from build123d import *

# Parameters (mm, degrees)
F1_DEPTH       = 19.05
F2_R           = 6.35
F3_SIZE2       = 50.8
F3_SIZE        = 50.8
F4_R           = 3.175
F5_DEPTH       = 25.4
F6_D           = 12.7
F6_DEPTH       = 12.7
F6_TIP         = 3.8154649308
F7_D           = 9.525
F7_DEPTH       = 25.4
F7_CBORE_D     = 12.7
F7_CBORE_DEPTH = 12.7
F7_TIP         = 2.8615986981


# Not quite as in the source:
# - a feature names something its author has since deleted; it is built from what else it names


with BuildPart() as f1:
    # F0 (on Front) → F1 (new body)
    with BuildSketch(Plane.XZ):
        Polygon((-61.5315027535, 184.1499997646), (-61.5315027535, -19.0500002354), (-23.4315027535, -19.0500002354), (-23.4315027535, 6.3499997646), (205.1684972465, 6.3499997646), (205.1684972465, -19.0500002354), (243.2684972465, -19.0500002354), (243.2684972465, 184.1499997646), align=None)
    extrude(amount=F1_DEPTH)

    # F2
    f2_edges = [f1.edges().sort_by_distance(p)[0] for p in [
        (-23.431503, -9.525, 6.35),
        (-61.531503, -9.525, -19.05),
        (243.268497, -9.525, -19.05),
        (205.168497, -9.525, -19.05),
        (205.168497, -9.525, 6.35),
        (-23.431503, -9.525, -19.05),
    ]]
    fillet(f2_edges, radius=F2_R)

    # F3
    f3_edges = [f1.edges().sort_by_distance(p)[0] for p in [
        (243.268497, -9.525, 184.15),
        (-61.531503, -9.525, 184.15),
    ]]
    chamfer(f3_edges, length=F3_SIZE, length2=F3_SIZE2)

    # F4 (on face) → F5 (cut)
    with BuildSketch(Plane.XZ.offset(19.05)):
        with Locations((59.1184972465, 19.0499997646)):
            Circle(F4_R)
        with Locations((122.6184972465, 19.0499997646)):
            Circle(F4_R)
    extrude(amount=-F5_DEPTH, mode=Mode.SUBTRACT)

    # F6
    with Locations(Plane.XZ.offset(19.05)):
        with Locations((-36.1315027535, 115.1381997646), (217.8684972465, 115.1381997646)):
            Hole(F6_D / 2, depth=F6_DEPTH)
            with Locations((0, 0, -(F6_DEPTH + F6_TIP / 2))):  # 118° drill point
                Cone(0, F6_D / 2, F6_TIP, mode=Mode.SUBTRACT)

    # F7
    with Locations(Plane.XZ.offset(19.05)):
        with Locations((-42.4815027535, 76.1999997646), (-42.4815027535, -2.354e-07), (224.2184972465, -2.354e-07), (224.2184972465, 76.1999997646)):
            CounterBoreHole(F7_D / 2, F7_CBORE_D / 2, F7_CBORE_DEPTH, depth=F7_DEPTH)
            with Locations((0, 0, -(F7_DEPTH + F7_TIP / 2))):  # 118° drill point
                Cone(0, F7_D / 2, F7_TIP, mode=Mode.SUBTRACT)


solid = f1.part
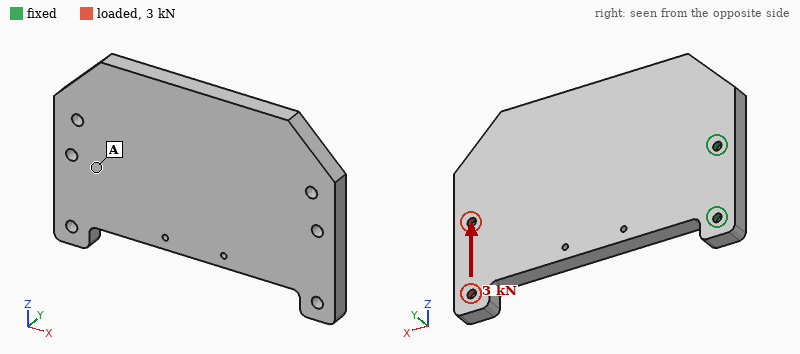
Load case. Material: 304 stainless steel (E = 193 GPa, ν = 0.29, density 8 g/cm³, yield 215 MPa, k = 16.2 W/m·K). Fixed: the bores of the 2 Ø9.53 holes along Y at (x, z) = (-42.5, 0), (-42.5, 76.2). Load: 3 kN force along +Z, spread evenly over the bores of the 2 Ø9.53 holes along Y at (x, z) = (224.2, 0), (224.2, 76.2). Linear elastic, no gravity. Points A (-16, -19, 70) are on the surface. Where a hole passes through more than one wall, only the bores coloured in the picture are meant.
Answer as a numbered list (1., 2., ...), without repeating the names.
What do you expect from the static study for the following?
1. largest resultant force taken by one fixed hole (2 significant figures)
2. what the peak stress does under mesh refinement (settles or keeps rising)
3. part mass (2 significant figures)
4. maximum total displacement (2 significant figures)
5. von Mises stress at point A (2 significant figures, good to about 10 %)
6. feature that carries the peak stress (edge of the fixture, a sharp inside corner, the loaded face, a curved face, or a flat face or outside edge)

1. 10 kN
2. keeps rising
3. 8.1 kg
4. 0.10 mm
5. 7.9 MPa
6. edge of the fixture
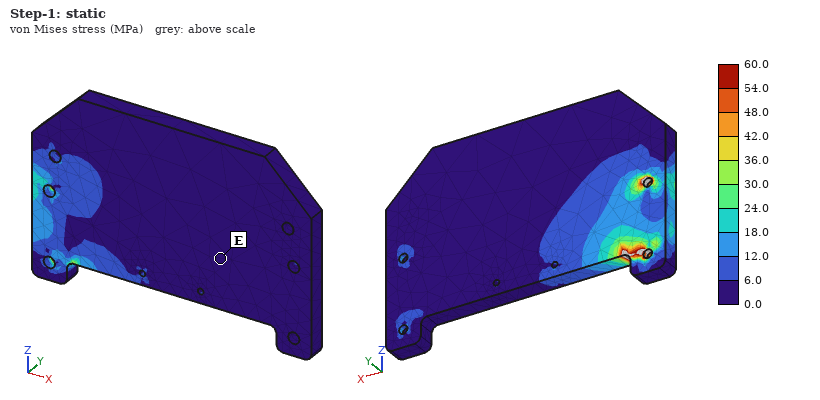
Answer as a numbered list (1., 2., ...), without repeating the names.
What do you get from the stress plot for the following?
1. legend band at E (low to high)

1. 0.0 to 6.0 MPa
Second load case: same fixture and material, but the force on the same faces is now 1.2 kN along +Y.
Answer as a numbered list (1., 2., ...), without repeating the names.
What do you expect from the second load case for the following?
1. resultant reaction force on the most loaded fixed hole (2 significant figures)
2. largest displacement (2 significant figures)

1. 1.6 kN
2. 1.1 mm
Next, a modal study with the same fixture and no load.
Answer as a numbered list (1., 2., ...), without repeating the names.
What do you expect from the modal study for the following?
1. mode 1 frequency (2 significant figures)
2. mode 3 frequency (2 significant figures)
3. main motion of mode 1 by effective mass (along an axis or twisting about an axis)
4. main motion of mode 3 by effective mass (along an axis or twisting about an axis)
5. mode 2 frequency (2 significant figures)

1. 110 Hz
2. 590 Hz
3. along Y
4. along Z
5. 450 Hz
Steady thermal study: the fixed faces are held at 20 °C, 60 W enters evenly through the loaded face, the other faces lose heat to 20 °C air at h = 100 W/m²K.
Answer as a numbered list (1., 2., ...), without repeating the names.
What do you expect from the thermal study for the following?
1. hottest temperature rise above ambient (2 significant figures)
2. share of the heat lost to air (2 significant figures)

1. 81 K
2. 100 %
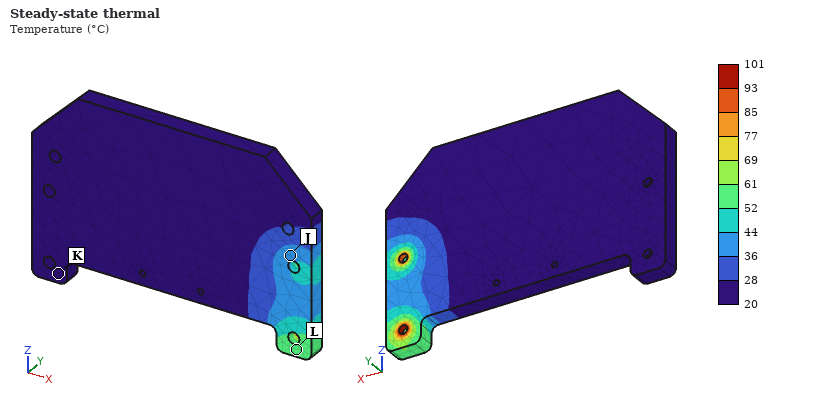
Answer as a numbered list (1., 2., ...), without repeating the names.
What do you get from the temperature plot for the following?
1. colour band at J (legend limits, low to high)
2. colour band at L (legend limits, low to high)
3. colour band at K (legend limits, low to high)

1. 36 to 44 °C
2. 52 to 61 °C
3. 20 to 28 °C
